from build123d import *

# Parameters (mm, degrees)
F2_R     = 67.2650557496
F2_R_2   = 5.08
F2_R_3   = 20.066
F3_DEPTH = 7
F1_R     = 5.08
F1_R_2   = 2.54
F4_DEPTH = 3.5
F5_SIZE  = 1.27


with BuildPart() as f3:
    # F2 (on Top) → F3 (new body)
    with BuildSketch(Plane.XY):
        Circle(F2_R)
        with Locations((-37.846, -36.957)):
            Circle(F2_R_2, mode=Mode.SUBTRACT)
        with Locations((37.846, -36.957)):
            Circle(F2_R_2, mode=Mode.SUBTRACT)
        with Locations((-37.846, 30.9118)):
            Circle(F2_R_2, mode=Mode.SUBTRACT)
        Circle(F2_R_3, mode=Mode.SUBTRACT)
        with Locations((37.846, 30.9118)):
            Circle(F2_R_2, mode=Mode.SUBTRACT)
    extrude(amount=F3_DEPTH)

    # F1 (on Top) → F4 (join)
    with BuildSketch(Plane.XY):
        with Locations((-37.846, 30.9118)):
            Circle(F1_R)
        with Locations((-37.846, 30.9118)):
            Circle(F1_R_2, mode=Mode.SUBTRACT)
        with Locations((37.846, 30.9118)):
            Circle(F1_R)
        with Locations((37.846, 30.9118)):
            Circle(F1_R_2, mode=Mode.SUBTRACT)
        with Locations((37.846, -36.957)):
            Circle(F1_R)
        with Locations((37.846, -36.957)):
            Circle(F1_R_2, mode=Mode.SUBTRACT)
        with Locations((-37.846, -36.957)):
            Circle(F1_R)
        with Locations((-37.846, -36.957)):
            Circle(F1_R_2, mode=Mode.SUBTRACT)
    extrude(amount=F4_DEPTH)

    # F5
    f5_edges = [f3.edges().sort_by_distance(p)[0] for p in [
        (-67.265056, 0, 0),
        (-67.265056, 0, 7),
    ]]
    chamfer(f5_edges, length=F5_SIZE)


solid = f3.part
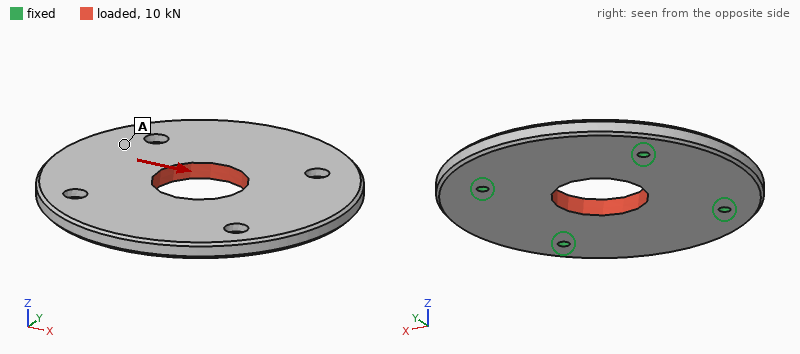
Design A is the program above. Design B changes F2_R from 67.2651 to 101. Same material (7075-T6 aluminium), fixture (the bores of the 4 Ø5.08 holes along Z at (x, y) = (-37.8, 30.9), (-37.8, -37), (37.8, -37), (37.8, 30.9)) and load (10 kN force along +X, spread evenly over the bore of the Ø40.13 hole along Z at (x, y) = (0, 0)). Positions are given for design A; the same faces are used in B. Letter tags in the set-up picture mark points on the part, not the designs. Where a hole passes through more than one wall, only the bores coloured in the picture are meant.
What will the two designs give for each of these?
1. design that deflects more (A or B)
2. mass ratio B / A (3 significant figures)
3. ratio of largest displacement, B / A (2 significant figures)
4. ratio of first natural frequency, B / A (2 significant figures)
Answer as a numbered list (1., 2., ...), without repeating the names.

1. B
2. 2.41
3. 1.6
4. 0.39
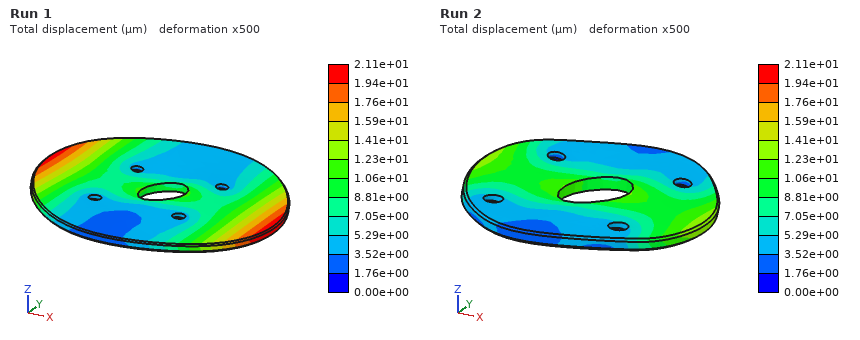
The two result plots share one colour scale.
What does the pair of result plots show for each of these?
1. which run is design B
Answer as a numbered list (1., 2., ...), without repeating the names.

1. Run 1
